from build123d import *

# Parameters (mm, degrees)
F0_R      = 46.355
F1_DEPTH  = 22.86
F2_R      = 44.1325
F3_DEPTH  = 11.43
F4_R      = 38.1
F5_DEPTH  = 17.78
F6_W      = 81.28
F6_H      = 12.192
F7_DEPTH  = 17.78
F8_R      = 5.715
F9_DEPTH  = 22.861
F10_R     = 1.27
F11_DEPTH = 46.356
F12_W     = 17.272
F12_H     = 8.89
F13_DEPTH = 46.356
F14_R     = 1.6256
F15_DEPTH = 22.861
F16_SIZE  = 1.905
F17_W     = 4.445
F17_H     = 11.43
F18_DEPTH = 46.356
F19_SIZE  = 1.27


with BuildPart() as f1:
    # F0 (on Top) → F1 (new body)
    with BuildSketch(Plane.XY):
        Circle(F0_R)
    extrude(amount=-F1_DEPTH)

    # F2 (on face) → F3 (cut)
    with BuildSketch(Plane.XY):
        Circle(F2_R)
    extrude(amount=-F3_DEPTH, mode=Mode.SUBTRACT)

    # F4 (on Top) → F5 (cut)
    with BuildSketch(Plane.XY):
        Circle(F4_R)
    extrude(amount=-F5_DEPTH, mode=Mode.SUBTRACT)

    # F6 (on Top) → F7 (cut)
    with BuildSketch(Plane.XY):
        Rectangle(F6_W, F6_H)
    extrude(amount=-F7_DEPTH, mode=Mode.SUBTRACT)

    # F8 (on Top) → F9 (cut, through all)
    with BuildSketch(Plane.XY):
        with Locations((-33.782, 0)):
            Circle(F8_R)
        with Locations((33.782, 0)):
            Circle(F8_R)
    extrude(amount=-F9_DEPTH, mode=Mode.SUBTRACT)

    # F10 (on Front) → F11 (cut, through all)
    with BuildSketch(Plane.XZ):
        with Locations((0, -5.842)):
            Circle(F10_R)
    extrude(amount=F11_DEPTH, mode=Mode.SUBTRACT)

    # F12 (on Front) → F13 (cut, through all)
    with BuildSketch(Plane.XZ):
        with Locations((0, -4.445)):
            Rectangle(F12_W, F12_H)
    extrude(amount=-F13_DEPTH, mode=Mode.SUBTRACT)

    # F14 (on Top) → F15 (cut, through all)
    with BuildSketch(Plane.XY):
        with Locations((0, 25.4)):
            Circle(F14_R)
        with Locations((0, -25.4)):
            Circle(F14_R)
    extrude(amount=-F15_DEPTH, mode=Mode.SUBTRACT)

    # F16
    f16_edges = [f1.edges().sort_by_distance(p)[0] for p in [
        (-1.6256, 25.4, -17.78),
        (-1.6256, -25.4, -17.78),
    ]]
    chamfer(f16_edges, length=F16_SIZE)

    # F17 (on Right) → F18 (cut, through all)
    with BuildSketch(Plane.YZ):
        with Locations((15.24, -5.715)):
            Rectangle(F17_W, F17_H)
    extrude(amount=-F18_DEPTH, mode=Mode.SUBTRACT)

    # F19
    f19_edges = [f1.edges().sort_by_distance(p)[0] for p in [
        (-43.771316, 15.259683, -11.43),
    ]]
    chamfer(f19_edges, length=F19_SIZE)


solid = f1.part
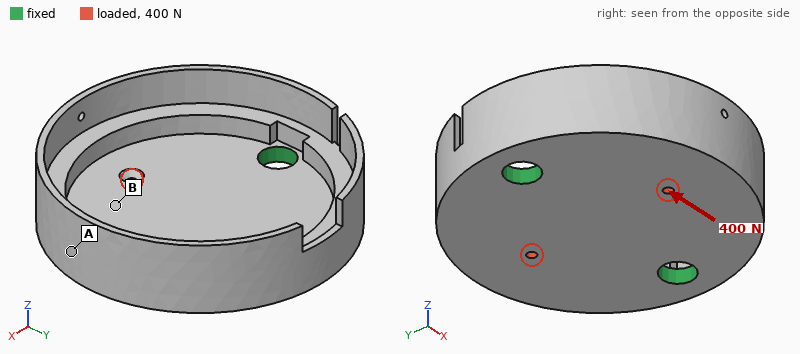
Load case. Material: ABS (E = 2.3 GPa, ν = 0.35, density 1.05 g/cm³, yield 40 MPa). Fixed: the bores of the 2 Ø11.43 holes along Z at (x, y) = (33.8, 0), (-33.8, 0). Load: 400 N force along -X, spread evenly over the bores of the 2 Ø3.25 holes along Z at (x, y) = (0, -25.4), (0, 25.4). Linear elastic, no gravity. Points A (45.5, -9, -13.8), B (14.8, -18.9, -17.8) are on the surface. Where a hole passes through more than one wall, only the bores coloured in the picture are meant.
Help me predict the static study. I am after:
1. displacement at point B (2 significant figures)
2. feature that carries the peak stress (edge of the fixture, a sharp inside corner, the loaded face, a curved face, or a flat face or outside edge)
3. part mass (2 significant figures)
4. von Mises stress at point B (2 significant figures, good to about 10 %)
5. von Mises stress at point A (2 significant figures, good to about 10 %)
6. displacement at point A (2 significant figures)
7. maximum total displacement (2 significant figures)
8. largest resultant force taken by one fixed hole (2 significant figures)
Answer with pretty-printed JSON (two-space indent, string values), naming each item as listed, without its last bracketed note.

{
  "displacement at point B": "13 µm",
  "feature that carries the peak stress": "the loaded face",
  "part mass": "56 g",
  "von Mises stress at point B": "1.1 MPa",
  "von Mises stress at point A": "0.46 MPa",
  "displacement at point A": "6.6 µm",
  "maximum total displacement": "30 µm",
  "largest resultant force taken by one fixed hole": "200 N"
}
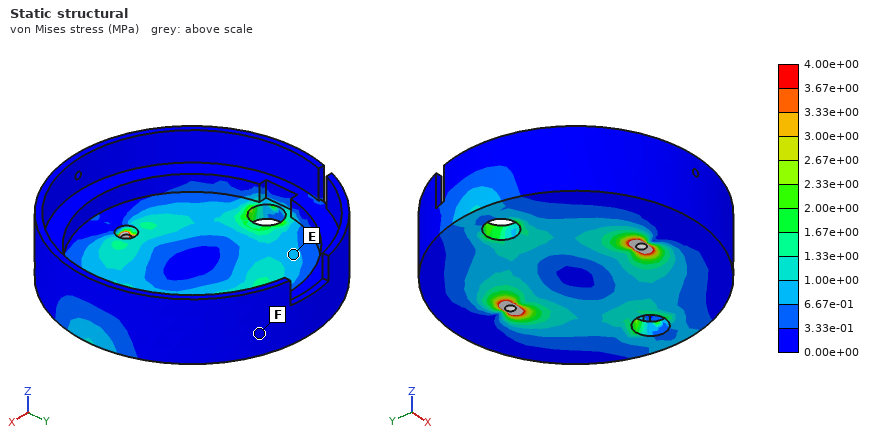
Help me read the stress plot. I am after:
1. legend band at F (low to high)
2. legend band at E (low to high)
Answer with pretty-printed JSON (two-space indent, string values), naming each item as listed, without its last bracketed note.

{
  "legend band at F": "0.00e+00 to 3.33e-01 MPa",
  "legend band at E": "6.67e-01 to 1.00e+00 MPa"
}
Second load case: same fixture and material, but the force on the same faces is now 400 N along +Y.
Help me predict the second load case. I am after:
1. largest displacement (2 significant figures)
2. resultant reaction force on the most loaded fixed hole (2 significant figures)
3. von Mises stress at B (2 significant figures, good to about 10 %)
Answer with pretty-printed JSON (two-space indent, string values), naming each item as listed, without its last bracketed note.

{
  "largest displacement": "43 µm",
  "resultant reaction force on the most loaded fixed hole": "200 N",
  "von Mises stress at B": "0.89 MPa"
}
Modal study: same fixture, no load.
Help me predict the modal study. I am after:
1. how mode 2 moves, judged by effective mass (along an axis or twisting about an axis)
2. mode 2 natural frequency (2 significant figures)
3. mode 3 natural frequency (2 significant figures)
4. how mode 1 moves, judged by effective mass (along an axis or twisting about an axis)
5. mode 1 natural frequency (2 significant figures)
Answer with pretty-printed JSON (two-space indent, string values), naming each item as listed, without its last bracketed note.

{
  "how mode 2 moves, judged by effective mass": "along Z",
  "mode 2 natural frequency": "940 Hz",
  "mode 3 natural frequency": "1500 Hz",
  "how mode 1 moves, judged by effective mass": "twisting about X",
  "mode 1 natural frequency": "750 Hz"
}
